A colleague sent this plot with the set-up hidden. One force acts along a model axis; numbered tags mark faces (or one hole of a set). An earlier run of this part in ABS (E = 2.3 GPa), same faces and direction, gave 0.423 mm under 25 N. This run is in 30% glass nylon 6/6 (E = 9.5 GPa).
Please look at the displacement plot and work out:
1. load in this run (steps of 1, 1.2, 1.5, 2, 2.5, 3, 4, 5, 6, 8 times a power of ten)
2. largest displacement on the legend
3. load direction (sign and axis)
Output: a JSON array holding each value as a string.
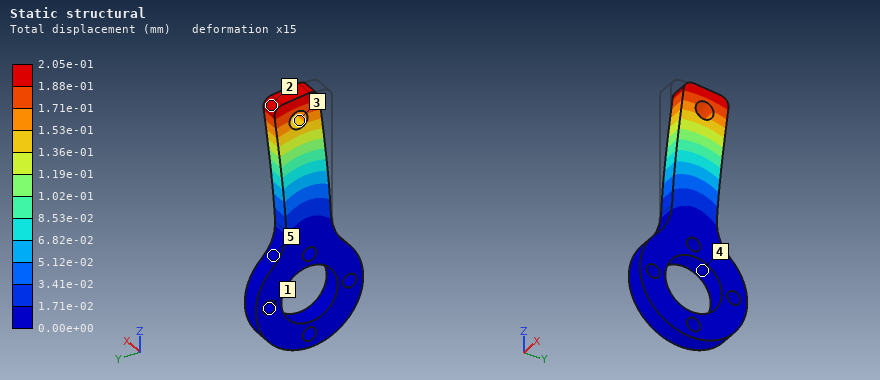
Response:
["50 N", "2.05e-01 mm", "+Y"]
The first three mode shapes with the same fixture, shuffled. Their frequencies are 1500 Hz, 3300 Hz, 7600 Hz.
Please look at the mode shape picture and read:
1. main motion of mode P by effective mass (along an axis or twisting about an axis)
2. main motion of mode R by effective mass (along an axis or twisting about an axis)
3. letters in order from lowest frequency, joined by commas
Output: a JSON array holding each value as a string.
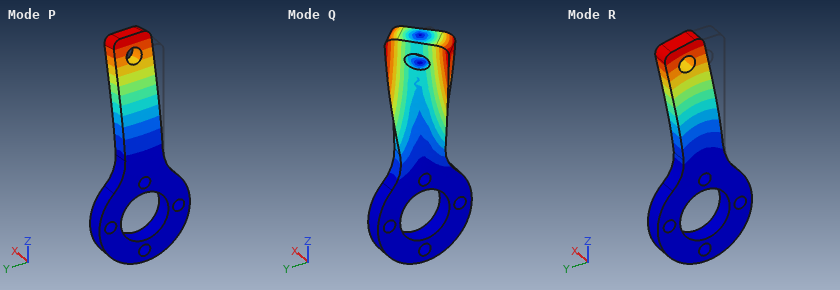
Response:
["along X", "along Y", "P, R, Q"]
